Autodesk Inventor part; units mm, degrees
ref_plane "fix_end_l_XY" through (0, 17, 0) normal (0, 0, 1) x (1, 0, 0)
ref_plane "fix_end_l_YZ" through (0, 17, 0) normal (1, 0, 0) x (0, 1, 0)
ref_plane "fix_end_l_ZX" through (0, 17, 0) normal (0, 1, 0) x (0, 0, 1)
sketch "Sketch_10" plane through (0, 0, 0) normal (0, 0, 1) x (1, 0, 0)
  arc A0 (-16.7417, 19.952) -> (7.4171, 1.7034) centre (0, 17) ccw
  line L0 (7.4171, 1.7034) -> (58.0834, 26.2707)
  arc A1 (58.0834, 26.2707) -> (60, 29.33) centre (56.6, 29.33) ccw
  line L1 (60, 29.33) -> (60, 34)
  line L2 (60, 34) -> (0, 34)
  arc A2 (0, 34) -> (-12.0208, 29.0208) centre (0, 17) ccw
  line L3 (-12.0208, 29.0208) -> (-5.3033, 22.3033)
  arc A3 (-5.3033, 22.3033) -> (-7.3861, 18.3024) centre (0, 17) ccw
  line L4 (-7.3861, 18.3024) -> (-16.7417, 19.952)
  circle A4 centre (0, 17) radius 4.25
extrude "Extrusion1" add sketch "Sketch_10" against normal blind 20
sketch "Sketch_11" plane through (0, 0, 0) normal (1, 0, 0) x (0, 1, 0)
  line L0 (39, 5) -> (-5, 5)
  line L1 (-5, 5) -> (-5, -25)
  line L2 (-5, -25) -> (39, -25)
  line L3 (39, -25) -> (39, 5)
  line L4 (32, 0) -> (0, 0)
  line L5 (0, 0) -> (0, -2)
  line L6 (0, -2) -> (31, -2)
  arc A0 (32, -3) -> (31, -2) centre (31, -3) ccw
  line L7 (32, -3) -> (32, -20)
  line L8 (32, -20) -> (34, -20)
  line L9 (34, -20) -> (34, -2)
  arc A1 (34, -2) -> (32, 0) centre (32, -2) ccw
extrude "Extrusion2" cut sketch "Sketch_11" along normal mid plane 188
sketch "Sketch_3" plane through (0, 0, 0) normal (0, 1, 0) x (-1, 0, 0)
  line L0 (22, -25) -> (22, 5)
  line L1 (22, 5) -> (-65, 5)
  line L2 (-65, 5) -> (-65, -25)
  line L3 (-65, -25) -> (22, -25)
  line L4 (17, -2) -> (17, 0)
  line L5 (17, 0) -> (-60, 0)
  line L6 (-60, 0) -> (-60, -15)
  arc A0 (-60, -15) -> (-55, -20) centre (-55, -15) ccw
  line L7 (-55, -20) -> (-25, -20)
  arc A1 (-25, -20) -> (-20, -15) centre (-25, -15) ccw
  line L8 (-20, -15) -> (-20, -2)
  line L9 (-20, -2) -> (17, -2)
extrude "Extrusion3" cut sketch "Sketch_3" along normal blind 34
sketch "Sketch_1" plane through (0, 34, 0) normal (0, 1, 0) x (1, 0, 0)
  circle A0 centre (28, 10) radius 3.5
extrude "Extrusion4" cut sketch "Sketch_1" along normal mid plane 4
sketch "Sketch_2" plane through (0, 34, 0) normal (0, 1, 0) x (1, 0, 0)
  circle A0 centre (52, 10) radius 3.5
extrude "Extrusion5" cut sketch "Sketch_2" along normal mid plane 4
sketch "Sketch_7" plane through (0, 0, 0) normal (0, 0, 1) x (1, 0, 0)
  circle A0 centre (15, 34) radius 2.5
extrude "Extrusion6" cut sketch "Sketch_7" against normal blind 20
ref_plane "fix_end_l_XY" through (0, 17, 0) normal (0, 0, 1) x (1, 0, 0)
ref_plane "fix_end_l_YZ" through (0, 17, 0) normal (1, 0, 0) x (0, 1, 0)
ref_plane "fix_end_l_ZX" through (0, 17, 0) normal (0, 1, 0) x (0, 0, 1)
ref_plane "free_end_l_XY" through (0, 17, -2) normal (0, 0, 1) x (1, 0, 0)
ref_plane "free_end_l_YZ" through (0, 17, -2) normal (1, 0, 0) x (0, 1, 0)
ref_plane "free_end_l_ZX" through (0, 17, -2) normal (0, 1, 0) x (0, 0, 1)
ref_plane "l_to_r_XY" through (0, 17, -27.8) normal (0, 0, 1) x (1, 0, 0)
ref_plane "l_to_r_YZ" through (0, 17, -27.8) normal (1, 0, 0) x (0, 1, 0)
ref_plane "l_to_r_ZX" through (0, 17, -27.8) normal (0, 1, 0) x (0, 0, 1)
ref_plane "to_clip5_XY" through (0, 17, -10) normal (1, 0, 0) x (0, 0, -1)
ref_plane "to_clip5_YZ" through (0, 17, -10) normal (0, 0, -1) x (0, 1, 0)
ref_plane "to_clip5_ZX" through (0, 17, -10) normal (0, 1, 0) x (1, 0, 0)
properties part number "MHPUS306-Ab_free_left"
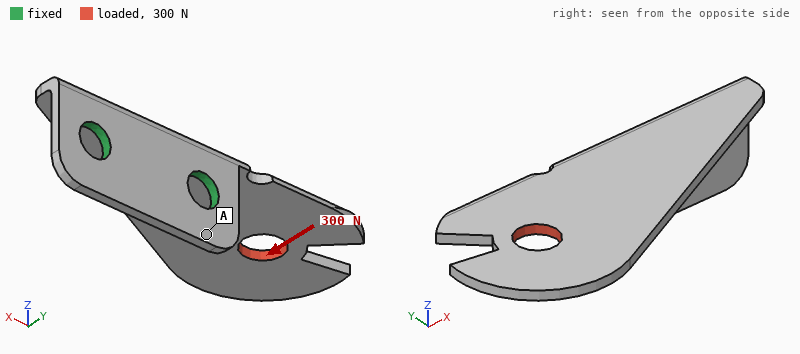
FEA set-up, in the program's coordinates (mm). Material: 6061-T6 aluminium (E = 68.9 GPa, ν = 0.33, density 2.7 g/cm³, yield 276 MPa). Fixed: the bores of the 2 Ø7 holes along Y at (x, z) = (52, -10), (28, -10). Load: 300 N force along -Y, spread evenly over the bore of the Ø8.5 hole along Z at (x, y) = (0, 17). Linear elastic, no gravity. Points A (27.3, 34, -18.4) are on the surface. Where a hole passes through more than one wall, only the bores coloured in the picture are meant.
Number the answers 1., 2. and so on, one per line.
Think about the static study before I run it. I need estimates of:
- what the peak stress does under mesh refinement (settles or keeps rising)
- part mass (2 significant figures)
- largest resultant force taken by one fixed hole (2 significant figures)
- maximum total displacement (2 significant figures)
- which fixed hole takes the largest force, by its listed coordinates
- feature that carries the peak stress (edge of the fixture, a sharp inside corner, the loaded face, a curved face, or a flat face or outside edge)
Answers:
1. keeps rising
2. 12 g
3. 620 N
4. 0.51 mm
5. (28, -10)
6. edge of the fixture
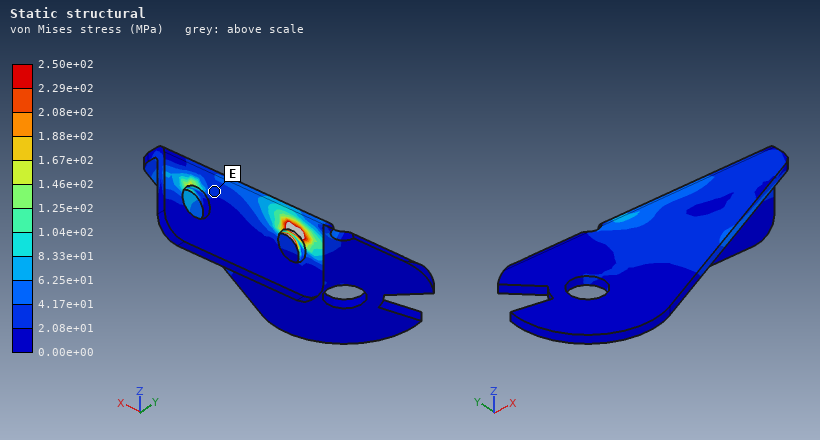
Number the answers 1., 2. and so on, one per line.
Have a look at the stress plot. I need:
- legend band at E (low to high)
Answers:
1. 2.08e+01 to 4.17e+01 MPa
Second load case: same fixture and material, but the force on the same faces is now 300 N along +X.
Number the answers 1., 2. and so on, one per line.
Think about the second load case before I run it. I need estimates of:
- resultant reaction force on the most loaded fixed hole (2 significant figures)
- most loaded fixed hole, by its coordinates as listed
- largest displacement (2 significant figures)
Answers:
1. 260 N
2. (52, -10)
3. 0.15 mm
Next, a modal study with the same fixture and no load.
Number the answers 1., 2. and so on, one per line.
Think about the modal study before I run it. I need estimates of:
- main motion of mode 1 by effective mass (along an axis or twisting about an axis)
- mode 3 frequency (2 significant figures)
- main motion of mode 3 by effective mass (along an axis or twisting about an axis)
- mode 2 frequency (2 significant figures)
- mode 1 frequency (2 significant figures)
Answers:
1. along Z
2. 2800 Hz
3. along Y
4. 1900 Hz
5. 700 Hz
